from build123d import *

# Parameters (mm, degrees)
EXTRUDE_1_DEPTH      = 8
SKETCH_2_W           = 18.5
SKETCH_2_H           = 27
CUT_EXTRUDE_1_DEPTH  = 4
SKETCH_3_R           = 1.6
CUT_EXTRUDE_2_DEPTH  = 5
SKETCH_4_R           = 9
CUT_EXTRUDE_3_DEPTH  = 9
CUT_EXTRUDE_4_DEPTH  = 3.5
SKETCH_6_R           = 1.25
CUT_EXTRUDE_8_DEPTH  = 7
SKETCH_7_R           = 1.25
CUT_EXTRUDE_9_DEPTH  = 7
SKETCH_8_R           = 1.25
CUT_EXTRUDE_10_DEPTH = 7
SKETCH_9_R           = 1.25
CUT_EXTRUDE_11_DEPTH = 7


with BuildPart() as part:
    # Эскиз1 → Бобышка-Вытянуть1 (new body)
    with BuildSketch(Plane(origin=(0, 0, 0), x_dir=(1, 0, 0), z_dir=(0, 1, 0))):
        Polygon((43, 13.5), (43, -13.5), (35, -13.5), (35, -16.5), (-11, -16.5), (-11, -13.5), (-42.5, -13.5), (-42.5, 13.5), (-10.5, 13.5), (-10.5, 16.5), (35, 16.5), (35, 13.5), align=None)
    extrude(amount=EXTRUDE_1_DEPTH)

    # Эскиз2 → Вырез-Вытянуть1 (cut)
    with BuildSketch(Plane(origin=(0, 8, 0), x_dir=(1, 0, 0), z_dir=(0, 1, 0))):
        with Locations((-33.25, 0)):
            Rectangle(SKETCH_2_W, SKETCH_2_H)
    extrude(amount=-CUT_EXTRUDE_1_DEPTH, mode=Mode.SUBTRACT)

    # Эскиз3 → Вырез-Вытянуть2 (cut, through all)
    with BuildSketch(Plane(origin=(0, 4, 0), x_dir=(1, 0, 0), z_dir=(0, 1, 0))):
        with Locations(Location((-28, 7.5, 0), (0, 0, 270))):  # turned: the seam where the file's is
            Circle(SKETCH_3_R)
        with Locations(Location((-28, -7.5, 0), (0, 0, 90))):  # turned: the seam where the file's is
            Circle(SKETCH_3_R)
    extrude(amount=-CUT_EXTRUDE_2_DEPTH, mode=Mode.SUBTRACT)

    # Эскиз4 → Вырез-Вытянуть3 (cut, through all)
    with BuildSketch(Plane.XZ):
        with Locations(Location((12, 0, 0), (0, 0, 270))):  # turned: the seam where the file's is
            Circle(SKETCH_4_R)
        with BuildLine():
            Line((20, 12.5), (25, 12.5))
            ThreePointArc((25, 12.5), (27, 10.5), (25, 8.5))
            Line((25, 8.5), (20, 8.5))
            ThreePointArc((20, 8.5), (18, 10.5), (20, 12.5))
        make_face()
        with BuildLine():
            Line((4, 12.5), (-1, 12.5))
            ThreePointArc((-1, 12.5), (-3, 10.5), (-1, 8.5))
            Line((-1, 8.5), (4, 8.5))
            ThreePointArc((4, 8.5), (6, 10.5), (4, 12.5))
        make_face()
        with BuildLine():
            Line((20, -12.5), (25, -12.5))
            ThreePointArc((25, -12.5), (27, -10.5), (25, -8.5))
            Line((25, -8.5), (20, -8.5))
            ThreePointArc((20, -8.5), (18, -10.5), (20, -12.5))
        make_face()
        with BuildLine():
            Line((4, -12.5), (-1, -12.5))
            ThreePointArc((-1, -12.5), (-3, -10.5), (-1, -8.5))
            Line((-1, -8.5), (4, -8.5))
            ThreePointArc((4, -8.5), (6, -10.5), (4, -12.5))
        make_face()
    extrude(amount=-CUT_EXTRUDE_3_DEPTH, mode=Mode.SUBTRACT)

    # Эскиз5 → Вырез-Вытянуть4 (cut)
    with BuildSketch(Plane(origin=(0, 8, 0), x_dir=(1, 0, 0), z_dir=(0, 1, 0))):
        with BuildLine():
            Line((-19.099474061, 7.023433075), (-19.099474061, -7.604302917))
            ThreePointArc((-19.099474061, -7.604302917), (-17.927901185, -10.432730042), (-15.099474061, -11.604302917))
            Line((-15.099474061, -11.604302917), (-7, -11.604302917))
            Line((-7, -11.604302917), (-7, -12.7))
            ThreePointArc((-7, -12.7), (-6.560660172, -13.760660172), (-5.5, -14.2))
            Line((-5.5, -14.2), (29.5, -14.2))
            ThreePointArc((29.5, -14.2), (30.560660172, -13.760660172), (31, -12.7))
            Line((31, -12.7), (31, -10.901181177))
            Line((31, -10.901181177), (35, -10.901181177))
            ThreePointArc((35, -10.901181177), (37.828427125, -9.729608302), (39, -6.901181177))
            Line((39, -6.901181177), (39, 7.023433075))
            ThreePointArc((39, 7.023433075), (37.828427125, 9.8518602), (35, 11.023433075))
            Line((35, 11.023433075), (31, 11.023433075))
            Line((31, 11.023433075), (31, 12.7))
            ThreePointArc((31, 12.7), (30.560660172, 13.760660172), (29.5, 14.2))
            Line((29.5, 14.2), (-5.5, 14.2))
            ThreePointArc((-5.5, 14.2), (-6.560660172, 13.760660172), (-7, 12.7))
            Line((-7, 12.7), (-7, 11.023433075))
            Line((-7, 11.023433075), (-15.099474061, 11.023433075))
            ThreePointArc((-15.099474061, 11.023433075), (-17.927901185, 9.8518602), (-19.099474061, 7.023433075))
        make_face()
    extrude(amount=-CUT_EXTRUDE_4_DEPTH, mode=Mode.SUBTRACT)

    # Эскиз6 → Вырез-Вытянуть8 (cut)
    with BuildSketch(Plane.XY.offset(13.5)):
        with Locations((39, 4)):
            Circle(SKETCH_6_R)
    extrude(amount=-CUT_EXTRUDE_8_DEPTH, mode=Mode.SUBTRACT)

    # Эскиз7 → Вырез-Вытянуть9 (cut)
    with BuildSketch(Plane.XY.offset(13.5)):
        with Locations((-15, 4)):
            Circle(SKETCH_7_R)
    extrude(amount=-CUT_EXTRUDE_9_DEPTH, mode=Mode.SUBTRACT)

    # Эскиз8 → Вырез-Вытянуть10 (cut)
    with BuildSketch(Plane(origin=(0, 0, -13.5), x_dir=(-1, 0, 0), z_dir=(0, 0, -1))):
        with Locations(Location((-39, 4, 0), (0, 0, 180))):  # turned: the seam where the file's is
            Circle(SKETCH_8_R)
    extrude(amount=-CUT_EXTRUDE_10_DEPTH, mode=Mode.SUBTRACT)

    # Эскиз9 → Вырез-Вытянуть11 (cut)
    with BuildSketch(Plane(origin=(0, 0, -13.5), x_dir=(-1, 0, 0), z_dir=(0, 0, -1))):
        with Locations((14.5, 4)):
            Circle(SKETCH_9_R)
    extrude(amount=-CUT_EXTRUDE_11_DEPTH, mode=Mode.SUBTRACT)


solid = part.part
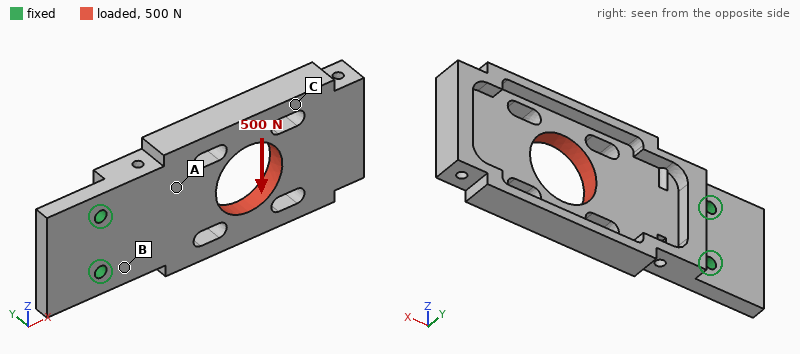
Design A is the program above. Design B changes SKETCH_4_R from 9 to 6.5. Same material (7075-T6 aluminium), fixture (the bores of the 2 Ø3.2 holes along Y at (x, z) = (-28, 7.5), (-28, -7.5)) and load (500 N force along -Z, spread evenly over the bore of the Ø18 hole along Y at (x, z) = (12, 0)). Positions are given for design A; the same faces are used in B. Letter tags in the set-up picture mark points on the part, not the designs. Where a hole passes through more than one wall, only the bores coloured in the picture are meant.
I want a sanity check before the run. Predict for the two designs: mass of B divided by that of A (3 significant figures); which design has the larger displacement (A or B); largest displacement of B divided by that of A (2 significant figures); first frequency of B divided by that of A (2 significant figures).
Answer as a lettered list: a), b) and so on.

a) 1.05
b) A
c) 0.91
d) 0.99
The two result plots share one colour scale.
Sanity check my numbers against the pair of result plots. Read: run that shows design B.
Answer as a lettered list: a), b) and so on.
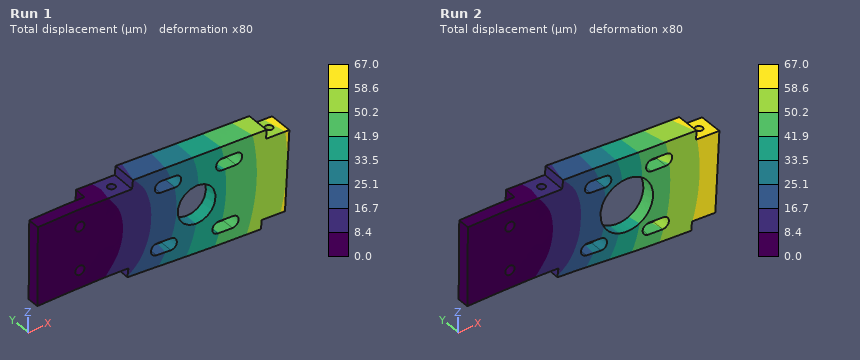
a) Run 1
